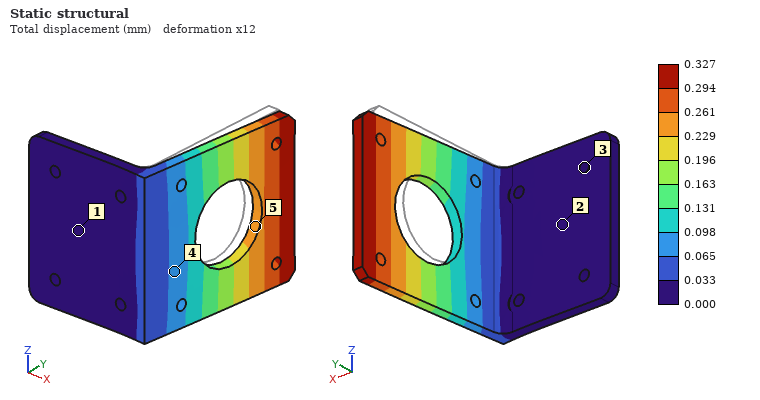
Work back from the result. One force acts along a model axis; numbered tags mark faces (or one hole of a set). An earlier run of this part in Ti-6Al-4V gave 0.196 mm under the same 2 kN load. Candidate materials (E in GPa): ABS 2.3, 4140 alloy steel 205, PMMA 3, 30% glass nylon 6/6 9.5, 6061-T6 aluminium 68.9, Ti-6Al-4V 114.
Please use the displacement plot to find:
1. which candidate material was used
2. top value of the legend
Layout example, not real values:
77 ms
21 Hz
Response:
6061-T6 aluminium
0.327 mm
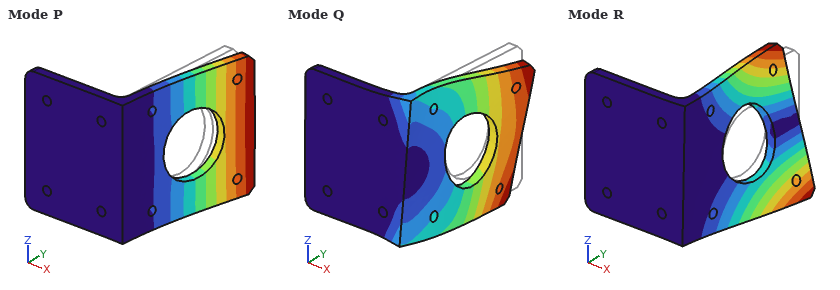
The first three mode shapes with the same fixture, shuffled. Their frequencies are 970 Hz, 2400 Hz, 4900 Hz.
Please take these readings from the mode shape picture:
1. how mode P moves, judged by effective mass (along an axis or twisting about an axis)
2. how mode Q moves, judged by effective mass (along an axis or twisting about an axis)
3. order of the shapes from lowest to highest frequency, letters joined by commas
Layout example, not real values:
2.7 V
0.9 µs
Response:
along X
along Z
P, R, Q
